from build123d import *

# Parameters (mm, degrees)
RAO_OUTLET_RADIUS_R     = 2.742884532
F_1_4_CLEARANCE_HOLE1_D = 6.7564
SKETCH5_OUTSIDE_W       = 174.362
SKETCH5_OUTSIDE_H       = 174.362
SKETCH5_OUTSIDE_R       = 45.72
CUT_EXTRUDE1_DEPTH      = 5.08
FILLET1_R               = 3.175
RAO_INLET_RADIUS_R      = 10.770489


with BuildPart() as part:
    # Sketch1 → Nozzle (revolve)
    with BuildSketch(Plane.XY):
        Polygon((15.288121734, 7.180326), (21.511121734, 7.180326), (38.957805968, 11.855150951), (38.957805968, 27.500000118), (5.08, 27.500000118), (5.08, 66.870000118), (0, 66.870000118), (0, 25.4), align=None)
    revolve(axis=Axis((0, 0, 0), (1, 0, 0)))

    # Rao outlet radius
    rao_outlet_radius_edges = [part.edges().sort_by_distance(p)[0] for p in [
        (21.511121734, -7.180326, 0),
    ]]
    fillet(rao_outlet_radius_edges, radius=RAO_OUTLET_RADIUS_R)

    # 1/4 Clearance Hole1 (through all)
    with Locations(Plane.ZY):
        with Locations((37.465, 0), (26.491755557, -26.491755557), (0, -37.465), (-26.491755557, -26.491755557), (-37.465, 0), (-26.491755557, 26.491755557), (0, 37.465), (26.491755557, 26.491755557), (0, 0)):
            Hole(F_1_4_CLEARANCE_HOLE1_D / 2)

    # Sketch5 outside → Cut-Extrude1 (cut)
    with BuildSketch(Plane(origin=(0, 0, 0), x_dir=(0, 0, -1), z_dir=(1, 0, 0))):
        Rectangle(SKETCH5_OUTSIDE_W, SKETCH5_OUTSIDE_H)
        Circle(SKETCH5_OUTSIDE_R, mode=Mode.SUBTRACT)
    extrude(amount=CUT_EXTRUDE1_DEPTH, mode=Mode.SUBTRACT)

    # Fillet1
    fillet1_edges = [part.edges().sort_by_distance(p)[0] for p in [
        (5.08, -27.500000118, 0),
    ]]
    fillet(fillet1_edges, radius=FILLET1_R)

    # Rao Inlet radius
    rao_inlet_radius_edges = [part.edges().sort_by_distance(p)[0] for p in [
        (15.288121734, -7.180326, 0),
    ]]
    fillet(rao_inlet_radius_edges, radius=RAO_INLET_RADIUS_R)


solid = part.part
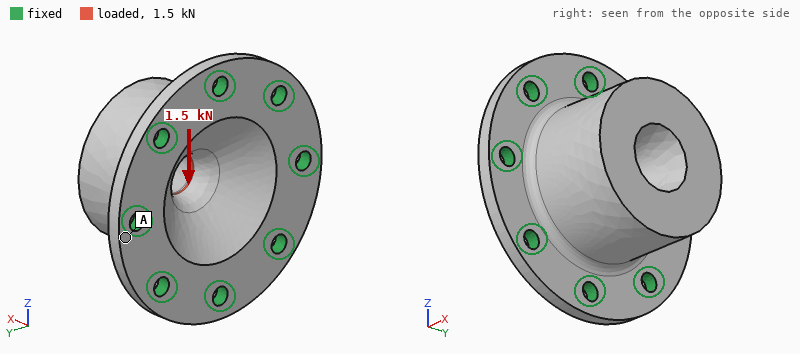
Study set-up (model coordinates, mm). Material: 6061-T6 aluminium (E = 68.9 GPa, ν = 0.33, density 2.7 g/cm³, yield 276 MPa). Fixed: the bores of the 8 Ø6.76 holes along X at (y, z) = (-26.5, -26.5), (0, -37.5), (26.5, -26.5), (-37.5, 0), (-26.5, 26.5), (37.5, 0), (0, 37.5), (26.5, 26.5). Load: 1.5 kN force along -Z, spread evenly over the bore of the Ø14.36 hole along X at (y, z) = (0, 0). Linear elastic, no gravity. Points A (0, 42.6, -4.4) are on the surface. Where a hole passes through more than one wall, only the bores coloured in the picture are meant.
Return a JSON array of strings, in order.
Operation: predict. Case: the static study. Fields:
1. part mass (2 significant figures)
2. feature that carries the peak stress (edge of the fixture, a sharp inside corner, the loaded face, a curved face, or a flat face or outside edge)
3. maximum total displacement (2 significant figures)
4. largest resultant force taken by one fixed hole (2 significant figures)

["250 g", "the loaded face", "3.5 µm", "360 N"]
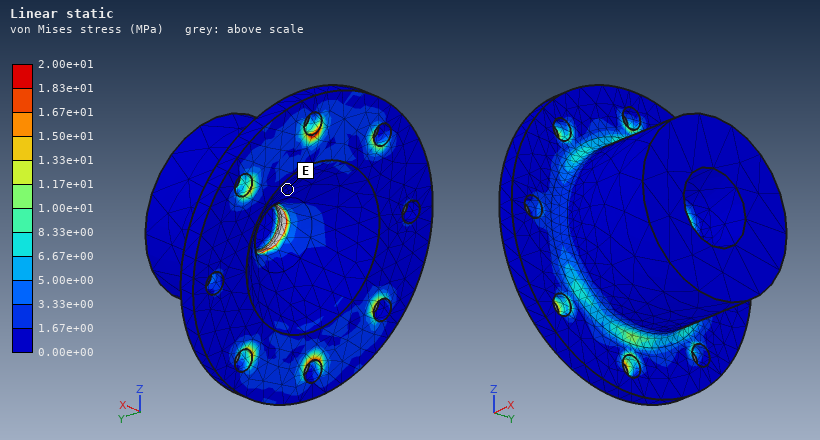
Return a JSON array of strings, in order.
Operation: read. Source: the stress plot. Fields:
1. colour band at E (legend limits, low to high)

["0.00e+00 to 1.67e+00 MPa"]
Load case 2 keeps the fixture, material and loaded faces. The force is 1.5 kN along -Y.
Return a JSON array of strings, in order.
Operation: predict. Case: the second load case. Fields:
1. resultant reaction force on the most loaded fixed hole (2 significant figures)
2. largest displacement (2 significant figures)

["360 N", "3.5 µm"]
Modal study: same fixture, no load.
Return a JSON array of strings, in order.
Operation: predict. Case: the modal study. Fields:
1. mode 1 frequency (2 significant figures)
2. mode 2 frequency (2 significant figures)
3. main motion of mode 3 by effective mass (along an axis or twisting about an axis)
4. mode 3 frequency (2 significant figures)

["8000 Hz", "8000 Hz", "along X", "9400 Hz"]
